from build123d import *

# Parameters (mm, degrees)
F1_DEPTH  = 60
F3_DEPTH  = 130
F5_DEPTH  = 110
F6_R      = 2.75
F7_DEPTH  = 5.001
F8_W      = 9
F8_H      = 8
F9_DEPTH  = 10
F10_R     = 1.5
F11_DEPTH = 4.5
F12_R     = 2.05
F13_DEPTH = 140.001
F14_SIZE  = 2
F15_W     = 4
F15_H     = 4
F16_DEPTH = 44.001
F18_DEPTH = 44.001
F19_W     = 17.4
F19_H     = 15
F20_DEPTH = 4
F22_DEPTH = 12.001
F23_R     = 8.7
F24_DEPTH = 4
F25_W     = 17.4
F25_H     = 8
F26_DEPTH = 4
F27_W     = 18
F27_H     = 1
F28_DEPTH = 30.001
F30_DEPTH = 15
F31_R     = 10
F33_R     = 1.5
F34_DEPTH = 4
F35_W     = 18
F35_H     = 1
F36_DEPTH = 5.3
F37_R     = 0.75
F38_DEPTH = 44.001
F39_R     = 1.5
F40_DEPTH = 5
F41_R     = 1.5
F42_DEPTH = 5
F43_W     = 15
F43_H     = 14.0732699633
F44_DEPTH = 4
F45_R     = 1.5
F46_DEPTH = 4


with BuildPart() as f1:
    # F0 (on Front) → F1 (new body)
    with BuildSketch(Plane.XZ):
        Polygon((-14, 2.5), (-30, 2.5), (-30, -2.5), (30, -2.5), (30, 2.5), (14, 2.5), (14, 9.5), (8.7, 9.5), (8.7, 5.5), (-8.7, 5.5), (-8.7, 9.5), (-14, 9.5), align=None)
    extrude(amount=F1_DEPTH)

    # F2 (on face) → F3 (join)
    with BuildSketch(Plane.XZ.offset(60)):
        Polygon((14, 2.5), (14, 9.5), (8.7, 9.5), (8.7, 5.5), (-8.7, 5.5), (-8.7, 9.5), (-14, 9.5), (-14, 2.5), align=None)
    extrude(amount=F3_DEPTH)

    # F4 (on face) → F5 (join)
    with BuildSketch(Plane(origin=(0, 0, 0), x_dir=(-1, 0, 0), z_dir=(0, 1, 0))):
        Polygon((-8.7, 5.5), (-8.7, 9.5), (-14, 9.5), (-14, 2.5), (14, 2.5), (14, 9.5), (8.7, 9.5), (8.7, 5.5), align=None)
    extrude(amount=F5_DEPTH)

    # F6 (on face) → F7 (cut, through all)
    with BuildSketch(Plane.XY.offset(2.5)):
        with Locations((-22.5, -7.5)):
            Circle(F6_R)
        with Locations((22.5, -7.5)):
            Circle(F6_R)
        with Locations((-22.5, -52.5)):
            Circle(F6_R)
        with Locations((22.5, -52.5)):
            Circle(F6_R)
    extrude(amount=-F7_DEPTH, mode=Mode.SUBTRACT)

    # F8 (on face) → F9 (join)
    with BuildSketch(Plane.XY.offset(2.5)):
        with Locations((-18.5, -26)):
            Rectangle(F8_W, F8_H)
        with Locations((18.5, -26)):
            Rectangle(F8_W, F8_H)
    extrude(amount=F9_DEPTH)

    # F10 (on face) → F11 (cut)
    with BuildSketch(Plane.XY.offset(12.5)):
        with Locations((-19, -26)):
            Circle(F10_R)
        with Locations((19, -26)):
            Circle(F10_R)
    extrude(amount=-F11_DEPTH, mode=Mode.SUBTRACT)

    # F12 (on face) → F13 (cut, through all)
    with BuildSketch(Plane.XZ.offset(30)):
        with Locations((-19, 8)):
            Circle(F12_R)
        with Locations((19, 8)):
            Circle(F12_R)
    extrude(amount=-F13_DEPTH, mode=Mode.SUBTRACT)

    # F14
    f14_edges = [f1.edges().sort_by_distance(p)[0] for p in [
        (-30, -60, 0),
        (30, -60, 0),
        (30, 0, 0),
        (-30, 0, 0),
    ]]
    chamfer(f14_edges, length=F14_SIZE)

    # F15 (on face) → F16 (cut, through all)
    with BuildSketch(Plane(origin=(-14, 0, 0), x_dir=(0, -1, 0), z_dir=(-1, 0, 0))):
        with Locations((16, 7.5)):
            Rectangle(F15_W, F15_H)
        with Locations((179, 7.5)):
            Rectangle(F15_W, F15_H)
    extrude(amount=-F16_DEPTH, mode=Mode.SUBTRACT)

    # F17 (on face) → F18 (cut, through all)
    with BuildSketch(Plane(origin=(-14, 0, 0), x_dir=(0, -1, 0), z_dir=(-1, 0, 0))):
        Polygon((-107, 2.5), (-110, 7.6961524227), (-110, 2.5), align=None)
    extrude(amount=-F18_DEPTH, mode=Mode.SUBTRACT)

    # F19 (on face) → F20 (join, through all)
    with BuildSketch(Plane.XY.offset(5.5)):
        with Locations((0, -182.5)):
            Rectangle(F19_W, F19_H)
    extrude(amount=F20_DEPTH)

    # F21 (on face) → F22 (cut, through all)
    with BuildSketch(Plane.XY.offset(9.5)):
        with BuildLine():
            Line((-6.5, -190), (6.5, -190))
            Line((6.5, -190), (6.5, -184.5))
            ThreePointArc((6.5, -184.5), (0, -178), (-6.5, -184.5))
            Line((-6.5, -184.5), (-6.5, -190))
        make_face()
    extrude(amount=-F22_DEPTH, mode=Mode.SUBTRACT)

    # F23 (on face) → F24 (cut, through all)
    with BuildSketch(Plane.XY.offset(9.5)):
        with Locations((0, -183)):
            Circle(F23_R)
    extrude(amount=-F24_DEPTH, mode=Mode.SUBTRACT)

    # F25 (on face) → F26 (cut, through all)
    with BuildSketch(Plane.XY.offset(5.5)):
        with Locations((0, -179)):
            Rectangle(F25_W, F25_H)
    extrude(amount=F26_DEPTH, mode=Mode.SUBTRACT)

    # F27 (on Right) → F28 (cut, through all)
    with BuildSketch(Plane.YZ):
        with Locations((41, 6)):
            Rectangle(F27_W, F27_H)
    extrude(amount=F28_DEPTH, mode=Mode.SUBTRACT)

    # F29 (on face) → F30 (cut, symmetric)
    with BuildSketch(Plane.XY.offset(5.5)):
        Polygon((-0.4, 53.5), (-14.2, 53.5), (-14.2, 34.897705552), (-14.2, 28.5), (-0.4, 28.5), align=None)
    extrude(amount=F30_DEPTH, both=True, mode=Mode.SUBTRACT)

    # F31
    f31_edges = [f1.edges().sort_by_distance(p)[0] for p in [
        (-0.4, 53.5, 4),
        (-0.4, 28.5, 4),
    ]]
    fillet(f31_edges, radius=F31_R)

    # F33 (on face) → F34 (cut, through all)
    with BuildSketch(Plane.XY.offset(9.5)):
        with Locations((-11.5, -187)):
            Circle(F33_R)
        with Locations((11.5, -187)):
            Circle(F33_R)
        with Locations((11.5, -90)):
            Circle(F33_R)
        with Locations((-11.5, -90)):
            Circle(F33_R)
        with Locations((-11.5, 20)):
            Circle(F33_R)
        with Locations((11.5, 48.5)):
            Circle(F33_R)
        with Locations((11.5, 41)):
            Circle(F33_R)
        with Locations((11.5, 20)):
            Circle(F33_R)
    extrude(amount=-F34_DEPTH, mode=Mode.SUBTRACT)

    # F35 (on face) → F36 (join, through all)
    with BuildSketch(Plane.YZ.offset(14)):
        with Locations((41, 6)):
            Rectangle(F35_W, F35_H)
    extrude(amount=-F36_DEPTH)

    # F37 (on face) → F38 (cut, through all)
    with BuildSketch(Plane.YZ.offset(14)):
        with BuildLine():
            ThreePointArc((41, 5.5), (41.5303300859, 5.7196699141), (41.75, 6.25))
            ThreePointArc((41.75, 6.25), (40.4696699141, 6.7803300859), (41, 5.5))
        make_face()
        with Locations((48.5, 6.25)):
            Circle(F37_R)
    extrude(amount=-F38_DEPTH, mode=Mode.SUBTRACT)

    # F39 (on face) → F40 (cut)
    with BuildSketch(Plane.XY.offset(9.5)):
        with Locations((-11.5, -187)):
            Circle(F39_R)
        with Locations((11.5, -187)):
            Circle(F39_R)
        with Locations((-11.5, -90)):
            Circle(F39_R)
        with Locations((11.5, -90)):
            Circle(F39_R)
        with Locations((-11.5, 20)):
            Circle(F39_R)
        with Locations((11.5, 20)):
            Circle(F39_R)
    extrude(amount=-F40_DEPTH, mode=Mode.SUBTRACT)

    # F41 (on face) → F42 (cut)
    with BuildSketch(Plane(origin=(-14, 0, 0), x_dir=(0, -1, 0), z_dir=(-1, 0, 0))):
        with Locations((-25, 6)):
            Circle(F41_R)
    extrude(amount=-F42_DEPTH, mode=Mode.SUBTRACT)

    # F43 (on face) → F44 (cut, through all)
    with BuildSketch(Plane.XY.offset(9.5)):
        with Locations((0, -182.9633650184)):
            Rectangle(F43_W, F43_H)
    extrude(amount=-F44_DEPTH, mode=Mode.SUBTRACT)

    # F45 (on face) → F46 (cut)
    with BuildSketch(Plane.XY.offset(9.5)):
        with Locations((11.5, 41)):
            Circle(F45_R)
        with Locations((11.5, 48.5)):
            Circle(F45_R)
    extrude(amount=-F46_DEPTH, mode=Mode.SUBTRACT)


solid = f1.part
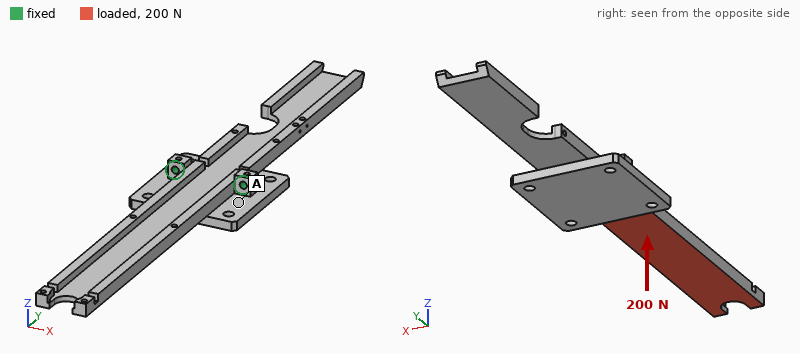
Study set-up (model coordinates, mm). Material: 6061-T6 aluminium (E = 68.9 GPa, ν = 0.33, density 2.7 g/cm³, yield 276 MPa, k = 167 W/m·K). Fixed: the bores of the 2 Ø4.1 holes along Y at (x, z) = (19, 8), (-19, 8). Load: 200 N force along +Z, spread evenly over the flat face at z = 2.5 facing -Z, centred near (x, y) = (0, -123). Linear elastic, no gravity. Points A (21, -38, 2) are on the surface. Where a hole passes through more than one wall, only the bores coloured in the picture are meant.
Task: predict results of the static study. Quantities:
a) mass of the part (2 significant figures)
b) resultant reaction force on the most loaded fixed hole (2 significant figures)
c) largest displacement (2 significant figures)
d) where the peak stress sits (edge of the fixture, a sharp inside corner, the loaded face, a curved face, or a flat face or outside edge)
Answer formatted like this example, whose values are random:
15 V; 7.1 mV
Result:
150 g; 180 N; 2.4 mm; a curved face
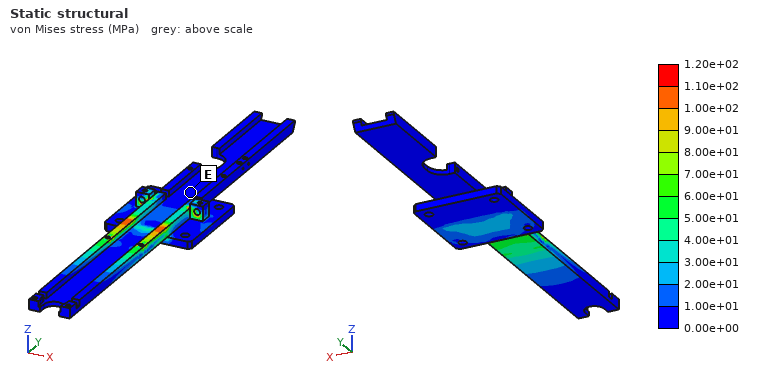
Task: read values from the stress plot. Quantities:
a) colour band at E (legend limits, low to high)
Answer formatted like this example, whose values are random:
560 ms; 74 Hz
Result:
0.00e+00 to 1.00e+01 MPa
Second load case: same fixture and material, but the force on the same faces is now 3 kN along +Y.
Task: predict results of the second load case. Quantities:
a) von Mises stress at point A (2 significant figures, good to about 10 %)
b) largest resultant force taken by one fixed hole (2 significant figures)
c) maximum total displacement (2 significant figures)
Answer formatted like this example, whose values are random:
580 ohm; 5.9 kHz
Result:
9.9 MPa; 1.5 kN; 1.6 mm
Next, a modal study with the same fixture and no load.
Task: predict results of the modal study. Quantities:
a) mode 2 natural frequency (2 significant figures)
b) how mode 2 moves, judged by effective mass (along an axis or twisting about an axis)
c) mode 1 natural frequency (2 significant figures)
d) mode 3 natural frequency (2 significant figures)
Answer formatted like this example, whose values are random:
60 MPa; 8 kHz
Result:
300 Hz; along Z; 280 Hz; 960 Hz
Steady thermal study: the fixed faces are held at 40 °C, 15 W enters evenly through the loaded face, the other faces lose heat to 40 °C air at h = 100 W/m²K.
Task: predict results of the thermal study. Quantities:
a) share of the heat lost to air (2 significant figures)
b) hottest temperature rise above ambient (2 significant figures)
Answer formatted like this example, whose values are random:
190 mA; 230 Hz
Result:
71 %; 17 K
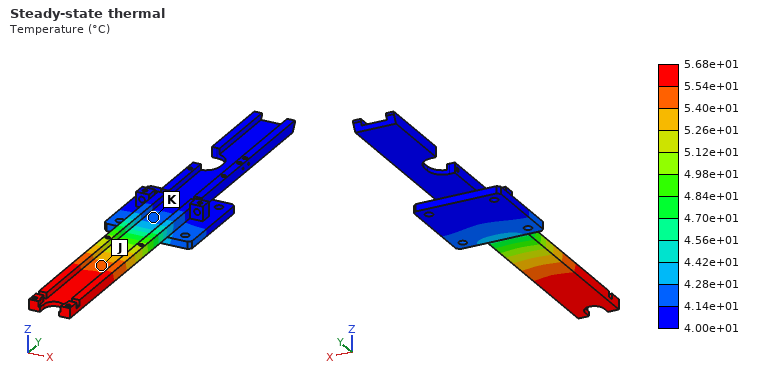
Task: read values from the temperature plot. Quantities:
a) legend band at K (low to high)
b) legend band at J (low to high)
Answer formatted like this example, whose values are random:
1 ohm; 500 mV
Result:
4.14e+01 to 4.28e+01 °C; 5.40e+01 to 5.54e+01 °C
